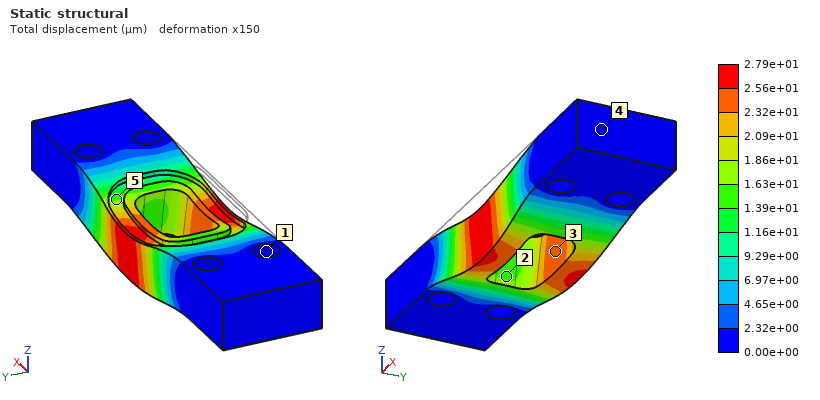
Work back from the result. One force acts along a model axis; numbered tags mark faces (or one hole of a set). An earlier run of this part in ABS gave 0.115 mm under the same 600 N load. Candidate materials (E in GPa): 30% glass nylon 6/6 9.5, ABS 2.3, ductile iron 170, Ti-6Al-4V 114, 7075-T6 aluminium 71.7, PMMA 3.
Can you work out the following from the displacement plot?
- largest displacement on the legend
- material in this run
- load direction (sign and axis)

2.79e+01 µm
30% glass nylon 6/6
-Z
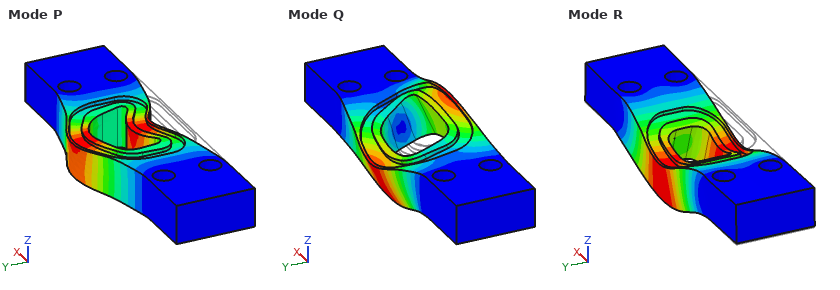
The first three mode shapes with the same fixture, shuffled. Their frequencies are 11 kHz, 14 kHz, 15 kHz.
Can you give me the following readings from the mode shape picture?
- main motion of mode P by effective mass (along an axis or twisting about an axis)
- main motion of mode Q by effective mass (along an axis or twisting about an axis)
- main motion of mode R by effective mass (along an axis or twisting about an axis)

along Y
twisting about X
along Z
